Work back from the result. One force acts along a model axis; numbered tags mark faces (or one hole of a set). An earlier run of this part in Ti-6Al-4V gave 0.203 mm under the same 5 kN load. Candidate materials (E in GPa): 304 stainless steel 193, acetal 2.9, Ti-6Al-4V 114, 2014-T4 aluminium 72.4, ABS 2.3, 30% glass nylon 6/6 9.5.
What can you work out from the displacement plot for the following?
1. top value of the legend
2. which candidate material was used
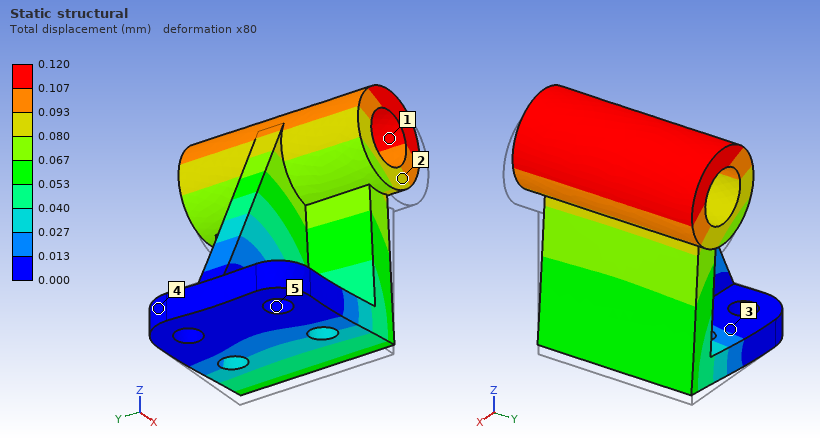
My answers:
0.120 mm
304 stainless steel
